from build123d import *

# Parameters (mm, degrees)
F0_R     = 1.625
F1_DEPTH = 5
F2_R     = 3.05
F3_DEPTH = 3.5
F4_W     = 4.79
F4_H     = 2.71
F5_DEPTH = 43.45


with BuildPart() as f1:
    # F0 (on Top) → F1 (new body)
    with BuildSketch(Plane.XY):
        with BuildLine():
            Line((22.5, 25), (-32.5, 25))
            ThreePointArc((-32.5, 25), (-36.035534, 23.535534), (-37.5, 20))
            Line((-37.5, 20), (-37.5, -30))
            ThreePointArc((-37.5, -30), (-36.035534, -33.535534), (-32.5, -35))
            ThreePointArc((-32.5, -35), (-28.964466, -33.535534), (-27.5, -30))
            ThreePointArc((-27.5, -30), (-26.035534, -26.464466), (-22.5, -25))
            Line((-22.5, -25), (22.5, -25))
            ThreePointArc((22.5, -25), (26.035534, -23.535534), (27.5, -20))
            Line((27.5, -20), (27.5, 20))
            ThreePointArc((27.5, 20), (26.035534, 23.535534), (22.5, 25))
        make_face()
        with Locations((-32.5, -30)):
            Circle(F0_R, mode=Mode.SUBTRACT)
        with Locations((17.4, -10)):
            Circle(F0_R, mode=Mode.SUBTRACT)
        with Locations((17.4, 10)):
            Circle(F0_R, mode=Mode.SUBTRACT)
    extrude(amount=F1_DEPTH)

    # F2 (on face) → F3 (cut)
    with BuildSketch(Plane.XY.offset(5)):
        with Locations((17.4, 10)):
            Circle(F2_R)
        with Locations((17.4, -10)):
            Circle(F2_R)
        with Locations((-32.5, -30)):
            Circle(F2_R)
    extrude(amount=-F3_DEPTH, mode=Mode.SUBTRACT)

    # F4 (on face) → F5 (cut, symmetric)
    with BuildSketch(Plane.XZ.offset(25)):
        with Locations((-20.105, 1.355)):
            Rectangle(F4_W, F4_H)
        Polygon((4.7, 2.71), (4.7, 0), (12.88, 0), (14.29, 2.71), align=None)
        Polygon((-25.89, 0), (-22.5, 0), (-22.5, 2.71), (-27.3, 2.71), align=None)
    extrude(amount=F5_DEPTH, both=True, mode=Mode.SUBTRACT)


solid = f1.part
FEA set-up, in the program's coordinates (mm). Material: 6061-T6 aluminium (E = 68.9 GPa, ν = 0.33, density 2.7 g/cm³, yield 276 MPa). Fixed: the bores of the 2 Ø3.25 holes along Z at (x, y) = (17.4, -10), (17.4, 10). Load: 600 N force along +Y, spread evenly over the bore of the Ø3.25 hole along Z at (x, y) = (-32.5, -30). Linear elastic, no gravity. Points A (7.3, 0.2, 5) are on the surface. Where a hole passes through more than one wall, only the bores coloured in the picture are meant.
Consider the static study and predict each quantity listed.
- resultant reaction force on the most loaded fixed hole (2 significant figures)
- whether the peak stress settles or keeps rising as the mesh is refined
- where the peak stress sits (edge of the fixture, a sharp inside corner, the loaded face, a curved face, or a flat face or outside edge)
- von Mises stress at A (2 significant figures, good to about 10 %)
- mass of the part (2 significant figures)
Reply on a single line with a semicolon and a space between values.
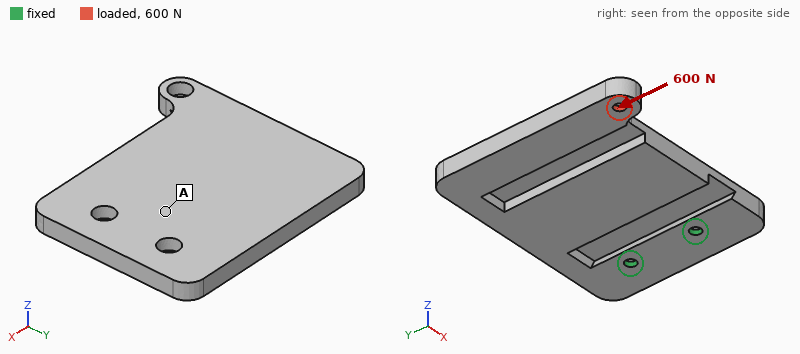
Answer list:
1.4 kN; keeps rising; edge of the fixture; 18 MPa; 38 g
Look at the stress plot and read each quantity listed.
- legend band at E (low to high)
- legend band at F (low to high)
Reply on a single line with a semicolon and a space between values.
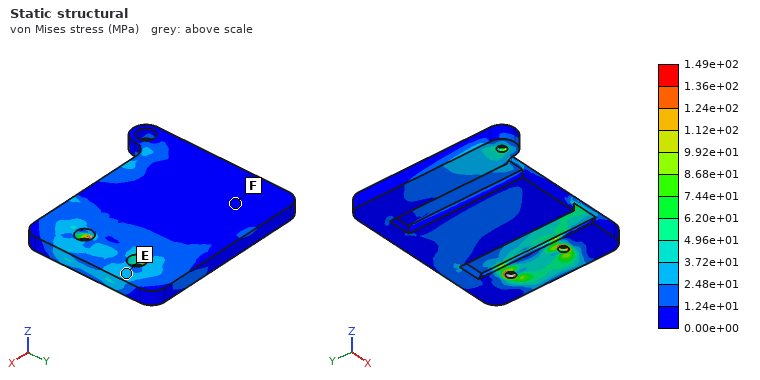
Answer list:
2.48e+01 to 3.72e+01 MPa; 0.00e+00 to 1.24e+01 MPa
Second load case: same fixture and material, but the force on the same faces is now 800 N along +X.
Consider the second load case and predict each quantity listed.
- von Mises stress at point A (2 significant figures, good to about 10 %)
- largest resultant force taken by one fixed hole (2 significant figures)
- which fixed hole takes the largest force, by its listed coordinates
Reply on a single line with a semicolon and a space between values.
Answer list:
35 MPa; 1.5 kN; (17.4, -10)
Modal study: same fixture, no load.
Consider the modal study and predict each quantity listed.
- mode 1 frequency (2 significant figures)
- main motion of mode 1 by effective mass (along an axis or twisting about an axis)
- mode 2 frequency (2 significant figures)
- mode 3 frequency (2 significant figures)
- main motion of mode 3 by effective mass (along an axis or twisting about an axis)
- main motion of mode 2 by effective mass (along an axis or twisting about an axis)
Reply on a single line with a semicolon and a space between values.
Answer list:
550 Hz; along Z; 2100 Hz; 3300 Hz; along Y; twisting about X
